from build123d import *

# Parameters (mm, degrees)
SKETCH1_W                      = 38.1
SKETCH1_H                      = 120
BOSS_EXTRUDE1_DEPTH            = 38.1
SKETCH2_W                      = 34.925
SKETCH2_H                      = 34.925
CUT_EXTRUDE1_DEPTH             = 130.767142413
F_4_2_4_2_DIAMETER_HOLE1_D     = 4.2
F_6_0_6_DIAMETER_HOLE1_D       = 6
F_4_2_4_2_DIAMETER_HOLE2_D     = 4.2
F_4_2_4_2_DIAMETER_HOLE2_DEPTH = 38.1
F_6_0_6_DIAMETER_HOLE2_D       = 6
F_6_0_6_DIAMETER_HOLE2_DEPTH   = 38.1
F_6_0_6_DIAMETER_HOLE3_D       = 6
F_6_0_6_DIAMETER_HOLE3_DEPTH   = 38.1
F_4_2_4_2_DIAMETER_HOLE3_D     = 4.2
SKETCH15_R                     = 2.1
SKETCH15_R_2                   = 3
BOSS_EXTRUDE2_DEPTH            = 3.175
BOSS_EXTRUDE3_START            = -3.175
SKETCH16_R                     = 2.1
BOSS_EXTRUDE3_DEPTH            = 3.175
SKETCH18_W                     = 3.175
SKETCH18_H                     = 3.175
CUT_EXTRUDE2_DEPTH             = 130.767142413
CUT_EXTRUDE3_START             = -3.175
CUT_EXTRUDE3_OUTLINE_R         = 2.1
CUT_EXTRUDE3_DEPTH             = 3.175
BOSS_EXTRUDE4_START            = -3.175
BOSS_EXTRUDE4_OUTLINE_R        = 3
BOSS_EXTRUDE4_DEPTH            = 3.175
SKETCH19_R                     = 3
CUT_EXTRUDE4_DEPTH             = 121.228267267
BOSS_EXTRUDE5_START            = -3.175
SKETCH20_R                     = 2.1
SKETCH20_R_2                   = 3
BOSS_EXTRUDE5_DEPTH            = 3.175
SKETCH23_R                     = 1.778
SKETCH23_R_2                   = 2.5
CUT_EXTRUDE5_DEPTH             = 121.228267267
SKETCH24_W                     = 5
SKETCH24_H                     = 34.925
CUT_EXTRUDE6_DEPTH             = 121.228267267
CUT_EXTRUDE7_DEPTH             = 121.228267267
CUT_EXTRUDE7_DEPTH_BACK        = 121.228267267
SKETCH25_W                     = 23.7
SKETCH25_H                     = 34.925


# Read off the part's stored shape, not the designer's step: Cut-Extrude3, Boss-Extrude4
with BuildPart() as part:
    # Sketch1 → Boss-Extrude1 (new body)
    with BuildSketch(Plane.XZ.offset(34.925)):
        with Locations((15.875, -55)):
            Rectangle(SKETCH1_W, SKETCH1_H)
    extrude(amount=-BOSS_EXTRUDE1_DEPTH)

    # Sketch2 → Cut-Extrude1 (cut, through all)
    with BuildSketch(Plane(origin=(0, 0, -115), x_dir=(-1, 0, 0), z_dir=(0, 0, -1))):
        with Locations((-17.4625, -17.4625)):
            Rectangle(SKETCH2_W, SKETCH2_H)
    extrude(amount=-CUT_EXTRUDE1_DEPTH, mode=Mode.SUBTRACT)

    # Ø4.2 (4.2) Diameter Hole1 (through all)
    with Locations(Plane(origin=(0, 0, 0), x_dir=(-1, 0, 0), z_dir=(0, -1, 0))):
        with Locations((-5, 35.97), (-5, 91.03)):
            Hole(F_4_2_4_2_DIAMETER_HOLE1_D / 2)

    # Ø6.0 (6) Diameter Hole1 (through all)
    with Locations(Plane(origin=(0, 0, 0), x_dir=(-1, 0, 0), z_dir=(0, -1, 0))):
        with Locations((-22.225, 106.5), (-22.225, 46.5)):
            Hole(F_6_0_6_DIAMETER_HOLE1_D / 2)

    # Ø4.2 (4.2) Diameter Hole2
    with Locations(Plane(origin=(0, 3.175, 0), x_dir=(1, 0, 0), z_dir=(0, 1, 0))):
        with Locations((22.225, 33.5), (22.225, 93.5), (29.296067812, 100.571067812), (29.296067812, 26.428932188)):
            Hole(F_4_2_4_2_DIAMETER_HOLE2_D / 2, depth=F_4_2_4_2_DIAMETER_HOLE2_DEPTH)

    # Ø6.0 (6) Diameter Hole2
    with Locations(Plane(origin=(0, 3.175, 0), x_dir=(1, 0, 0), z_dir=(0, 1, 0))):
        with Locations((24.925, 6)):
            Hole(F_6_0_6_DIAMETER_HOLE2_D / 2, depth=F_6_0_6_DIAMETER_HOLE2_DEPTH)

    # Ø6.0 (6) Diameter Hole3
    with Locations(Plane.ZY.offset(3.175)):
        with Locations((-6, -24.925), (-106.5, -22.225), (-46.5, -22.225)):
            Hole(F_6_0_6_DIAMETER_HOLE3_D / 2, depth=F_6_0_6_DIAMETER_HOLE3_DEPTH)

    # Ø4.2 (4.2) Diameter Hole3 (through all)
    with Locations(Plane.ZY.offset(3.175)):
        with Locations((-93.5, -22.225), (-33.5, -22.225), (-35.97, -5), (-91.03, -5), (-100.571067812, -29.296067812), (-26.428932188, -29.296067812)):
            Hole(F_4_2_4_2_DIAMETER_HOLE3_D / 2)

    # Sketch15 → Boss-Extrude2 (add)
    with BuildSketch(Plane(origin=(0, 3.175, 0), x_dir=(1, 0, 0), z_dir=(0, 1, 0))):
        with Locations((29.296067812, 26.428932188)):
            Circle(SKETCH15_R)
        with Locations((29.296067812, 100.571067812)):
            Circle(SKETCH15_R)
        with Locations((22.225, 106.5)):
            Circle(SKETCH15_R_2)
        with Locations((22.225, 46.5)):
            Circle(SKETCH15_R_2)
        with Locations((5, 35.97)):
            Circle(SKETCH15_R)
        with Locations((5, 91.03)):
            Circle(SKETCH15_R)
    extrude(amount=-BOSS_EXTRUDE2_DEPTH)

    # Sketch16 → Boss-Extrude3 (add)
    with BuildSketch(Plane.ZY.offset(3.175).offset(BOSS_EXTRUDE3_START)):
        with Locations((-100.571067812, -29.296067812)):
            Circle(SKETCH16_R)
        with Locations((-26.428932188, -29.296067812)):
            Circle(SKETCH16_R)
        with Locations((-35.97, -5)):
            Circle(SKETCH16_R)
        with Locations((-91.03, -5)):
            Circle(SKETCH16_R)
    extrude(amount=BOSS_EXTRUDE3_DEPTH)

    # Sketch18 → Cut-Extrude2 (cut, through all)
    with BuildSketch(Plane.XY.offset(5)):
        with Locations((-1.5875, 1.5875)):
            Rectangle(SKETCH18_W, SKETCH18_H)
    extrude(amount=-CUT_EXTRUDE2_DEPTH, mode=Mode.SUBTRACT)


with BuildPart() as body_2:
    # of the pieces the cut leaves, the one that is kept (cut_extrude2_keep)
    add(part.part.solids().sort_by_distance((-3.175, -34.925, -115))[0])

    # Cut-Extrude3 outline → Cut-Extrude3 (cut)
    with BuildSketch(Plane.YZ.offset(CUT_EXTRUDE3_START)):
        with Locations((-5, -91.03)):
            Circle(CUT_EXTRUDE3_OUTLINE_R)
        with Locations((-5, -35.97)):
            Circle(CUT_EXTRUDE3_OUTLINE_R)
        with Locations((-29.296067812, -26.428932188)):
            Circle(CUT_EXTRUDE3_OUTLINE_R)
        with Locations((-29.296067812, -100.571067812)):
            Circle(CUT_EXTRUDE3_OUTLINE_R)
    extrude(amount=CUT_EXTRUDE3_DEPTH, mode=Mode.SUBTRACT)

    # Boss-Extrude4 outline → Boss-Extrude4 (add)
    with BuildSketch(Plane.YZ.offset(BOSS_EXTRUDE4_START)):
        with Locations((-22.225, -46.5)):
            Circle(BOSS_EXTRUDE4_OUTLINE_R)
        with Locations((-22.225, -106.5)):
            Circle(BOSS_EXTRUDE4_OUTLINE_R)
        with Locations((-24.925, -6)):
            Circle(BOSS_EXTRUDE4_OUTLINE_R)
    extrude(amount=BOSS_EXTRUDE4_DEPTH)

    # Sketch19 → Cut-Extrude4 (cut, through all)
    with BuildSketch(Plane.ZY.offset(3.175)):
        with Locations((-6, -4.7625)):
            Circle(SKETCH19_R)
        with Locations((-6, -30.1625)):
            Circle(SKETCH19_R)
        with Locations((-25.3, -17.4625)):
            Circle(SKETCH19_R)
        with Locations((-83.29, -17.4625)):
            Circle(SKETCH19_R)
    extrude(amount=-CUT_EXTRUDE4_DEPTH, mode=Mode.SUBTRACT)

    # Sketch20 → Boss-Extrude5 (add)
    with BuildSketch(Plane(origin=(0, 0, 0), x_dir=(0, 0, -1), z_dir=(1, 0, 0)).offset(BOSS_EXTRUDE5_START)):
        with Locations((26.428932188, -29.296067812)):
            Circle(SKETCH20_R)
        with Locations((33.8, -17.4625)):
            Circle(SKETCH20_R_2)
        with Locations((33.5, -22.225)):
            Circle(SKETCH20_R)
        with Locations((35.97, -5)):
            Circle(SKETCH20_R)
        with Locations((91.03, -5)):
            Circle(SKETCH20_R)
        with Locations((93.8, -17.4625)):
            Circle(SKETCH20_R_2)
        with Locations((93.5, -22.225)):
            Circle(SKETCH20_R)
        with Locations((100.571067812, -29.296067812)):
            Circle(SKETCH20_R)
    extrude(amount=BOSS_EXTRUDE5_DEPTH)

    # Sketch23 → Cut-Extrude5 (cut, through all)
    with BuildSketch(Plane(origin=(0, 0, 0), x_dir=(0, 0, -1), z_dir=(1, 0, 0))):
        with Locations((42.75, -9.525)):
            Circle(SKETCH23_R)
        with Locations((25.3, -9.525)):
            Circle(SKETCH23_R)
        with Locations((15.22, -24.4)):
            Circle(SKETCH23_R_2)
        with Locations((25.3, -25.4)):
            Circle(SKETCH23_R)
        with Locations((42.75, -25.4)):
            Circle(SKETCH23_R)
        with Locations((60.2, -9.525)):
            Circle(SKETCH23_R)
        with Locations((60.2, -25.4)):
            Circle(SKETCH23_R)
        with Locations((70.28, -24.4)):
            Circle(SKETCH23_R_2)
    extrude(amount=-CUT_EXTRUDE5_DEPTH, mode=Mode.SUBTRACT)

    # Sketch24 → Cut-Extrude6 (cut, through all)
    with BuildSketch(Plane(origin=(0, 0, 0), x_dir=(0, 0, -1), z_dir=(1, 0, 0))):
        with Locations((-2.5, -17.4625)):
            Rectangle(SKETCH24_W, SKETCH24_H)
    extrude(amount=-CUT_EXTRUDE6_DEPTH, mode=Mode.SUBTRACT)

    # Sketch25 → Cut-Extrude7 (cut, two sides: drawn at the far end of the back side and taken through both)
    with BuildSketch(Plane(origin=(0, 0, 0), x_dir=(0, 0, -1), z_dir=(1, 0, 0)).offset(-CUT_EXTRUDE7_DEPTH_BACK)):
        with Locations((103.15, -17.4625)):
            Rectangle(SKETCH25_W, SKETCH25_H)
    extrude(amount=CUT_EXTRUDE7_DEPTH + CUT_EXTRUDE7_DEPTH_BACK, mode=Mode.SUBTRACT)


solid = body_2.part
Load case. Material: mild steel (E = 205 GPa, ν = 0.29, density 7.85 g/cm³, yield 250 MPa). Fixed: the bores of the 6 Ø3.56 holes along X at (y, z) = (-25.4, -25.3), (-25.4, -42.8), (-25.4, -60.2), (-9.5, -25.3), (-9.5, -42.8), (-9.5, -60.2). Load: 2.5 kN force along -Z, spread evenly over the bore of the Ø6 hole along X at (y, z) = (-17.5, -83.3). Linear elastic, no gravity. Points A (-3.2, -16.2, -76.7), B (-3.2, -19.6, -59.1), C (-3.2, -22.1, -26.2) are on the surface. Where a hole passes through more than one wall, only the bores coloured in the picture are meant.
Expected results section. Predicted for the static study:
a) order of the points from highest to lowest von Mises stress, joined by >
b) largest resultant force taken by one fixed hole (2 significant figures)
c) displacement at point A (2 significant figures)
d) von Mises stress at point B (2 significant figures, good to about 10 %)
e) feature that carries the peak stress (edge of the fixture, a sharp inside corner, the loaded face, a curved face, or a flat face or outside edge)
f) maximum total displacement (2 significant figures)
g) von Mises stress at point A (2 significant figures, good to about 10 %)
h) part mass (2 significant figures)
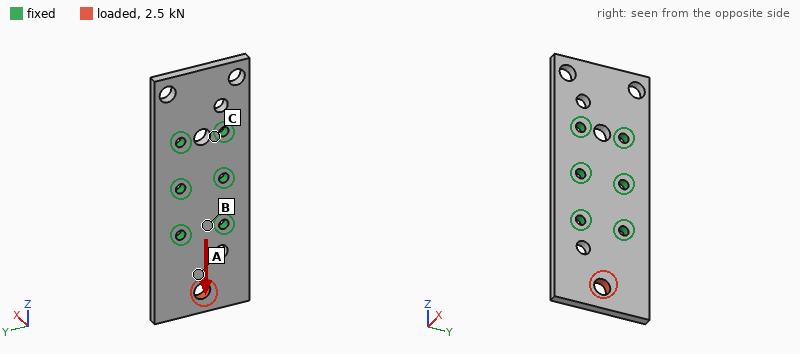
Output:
A > B > C
1.1 kN
3.0 µm
13 MPa
the loaded face
6.2 µm
47 MPa
74 g
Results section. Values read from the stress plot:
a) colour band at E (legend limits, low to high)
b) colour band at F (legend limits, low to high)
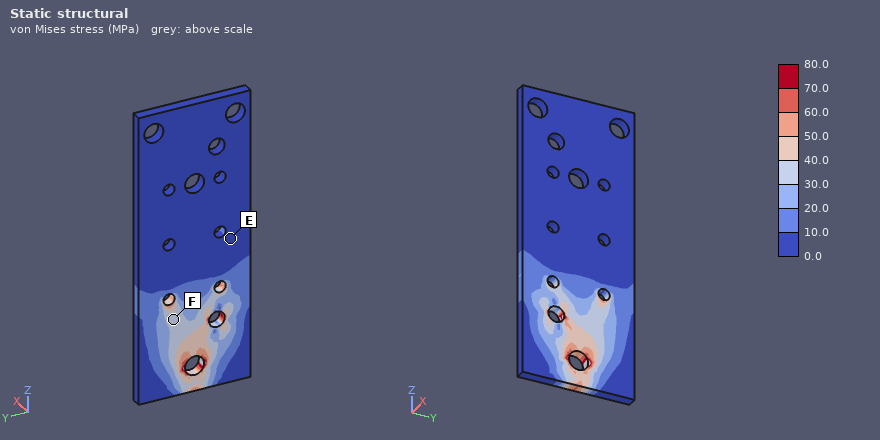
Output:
0.0 to 10.0 MPa
30.0 to 40.0 MPa
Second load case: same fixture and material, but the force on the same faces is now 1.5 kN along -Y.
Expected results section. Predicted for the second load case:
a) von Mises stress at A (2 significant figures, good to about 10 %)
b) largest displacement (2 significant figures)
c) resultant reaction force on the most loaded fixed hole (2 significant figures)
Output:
41 MPa
14 µm
1.5 kN
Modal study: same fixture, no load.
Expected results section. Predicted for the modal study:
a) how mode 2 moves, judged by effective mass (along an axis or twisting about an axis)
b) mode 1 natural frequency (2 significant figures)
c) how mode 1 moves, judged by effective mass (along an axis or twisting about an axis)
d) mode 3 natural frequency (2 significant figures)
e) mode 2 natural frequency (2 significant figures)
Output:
along X
2700 Hz
along X
5500 Hz
4200 Hz
